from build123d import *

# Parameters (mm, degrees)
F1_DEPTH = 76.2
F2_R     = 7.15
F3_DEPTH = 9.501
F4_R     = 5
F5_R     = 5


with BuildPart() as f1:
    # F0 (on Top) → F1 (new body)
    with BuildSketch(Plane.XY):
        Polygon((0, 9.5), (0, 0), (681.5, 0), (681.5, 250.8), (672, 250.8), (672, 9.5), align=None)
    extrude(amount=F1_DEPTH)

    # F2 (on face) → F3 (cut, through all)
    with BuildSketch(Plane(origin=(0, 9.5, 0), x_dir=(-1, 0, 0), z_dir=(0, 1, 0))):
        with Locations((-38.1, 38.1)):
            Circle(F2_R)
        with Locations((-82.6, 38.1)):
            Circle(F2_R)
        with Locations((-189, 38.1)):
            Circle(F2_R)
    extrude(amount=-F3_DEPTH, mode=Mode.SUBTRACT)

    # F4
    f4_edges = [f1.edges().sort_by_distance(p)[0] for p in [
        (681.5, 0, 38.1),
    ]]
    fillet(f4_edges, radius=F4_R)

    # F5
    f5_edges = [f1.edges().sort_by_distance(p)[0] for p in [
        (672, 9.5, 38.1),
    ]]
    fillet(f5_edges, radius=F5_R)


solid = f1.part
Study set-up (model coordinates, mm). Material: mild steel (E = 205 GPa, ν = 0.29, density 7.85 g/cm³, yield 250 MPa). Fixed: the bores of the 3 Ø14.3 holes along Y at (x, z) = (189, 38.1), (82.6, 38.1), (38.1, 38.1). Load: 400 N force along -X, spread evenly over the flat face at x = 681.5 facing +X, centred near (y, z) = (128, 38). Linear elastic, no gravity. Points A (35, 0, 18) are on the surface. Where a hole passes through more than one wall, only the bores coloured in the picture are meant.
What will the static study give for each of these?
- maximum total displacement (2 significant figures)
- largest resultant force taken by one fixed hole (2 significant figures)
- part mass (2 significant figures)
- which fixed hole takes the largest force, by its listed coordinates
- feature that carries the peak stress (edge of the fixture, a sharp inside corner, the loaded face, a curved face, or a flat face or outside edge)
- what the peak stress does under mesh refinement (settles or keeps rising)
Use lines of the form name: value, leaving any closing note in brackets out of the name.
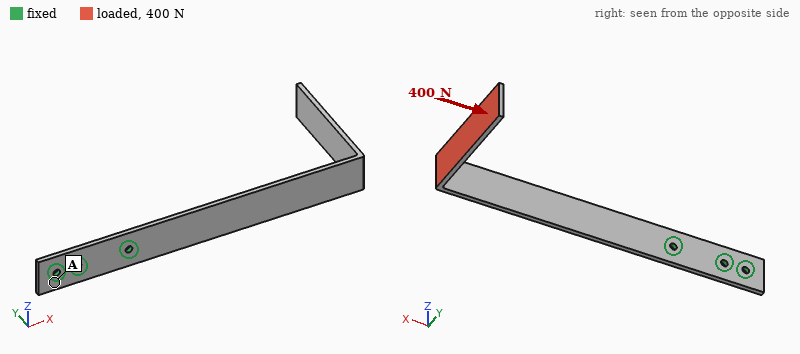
maximum total displacement: 7.9 mm
largest resultant force taken by one fixed hole: 350 N
part mass: 5.2 kg
which fixed hole takes the largest force, by its listed coordinates: (189, 38.1)
feature that carries the peak stress: edge of the fixture
what the peak stress does under mesh refinement: keeps rising
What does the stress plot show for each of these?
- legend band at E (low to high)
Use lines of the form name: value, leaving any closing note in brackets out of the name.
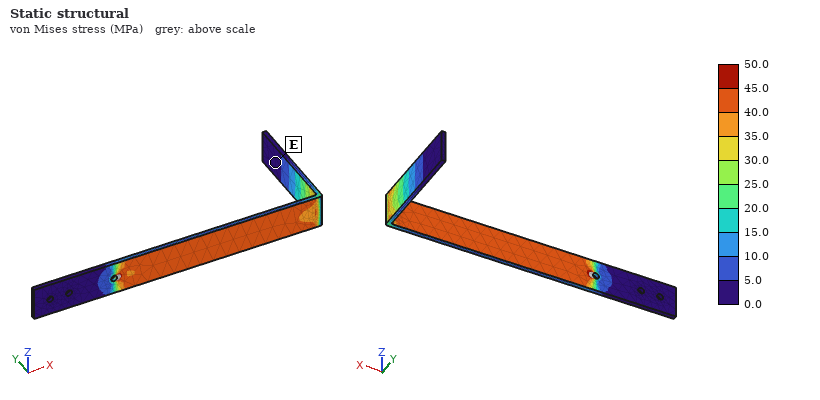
legend band at E: 0.0 to 5.0 MPa
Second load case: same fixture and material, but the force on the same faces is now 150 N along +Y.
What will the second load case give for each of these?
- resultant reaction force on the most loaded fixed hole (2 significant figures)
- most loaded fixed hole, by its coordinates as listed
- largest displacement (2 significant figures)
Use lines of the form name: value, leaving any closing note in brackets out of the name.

resultant reaction force on the most loaded fixed hole: 240 N
most loaded fixed hole, by its coordinates as listed: (189, 38.1)
largest displacement: 6.6 mm
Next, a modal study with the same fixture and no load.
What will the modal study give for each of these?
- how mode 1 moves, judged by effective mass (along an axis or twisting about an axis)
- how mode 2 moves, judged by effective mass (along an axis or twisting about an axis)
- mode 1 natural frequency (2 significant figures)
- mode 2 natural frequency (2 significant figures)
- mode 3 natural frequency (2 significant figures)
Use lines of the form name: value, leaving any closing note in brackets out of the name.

how mode 1 moves, judged by effective mass: along Y
how mode 2 moves, judged by effective mass: along Z
mode 1 natural frequency: 18 Hz
mode 2 natural frequency: 52 Hz
mode 3 natural frequency: 73 Hz
